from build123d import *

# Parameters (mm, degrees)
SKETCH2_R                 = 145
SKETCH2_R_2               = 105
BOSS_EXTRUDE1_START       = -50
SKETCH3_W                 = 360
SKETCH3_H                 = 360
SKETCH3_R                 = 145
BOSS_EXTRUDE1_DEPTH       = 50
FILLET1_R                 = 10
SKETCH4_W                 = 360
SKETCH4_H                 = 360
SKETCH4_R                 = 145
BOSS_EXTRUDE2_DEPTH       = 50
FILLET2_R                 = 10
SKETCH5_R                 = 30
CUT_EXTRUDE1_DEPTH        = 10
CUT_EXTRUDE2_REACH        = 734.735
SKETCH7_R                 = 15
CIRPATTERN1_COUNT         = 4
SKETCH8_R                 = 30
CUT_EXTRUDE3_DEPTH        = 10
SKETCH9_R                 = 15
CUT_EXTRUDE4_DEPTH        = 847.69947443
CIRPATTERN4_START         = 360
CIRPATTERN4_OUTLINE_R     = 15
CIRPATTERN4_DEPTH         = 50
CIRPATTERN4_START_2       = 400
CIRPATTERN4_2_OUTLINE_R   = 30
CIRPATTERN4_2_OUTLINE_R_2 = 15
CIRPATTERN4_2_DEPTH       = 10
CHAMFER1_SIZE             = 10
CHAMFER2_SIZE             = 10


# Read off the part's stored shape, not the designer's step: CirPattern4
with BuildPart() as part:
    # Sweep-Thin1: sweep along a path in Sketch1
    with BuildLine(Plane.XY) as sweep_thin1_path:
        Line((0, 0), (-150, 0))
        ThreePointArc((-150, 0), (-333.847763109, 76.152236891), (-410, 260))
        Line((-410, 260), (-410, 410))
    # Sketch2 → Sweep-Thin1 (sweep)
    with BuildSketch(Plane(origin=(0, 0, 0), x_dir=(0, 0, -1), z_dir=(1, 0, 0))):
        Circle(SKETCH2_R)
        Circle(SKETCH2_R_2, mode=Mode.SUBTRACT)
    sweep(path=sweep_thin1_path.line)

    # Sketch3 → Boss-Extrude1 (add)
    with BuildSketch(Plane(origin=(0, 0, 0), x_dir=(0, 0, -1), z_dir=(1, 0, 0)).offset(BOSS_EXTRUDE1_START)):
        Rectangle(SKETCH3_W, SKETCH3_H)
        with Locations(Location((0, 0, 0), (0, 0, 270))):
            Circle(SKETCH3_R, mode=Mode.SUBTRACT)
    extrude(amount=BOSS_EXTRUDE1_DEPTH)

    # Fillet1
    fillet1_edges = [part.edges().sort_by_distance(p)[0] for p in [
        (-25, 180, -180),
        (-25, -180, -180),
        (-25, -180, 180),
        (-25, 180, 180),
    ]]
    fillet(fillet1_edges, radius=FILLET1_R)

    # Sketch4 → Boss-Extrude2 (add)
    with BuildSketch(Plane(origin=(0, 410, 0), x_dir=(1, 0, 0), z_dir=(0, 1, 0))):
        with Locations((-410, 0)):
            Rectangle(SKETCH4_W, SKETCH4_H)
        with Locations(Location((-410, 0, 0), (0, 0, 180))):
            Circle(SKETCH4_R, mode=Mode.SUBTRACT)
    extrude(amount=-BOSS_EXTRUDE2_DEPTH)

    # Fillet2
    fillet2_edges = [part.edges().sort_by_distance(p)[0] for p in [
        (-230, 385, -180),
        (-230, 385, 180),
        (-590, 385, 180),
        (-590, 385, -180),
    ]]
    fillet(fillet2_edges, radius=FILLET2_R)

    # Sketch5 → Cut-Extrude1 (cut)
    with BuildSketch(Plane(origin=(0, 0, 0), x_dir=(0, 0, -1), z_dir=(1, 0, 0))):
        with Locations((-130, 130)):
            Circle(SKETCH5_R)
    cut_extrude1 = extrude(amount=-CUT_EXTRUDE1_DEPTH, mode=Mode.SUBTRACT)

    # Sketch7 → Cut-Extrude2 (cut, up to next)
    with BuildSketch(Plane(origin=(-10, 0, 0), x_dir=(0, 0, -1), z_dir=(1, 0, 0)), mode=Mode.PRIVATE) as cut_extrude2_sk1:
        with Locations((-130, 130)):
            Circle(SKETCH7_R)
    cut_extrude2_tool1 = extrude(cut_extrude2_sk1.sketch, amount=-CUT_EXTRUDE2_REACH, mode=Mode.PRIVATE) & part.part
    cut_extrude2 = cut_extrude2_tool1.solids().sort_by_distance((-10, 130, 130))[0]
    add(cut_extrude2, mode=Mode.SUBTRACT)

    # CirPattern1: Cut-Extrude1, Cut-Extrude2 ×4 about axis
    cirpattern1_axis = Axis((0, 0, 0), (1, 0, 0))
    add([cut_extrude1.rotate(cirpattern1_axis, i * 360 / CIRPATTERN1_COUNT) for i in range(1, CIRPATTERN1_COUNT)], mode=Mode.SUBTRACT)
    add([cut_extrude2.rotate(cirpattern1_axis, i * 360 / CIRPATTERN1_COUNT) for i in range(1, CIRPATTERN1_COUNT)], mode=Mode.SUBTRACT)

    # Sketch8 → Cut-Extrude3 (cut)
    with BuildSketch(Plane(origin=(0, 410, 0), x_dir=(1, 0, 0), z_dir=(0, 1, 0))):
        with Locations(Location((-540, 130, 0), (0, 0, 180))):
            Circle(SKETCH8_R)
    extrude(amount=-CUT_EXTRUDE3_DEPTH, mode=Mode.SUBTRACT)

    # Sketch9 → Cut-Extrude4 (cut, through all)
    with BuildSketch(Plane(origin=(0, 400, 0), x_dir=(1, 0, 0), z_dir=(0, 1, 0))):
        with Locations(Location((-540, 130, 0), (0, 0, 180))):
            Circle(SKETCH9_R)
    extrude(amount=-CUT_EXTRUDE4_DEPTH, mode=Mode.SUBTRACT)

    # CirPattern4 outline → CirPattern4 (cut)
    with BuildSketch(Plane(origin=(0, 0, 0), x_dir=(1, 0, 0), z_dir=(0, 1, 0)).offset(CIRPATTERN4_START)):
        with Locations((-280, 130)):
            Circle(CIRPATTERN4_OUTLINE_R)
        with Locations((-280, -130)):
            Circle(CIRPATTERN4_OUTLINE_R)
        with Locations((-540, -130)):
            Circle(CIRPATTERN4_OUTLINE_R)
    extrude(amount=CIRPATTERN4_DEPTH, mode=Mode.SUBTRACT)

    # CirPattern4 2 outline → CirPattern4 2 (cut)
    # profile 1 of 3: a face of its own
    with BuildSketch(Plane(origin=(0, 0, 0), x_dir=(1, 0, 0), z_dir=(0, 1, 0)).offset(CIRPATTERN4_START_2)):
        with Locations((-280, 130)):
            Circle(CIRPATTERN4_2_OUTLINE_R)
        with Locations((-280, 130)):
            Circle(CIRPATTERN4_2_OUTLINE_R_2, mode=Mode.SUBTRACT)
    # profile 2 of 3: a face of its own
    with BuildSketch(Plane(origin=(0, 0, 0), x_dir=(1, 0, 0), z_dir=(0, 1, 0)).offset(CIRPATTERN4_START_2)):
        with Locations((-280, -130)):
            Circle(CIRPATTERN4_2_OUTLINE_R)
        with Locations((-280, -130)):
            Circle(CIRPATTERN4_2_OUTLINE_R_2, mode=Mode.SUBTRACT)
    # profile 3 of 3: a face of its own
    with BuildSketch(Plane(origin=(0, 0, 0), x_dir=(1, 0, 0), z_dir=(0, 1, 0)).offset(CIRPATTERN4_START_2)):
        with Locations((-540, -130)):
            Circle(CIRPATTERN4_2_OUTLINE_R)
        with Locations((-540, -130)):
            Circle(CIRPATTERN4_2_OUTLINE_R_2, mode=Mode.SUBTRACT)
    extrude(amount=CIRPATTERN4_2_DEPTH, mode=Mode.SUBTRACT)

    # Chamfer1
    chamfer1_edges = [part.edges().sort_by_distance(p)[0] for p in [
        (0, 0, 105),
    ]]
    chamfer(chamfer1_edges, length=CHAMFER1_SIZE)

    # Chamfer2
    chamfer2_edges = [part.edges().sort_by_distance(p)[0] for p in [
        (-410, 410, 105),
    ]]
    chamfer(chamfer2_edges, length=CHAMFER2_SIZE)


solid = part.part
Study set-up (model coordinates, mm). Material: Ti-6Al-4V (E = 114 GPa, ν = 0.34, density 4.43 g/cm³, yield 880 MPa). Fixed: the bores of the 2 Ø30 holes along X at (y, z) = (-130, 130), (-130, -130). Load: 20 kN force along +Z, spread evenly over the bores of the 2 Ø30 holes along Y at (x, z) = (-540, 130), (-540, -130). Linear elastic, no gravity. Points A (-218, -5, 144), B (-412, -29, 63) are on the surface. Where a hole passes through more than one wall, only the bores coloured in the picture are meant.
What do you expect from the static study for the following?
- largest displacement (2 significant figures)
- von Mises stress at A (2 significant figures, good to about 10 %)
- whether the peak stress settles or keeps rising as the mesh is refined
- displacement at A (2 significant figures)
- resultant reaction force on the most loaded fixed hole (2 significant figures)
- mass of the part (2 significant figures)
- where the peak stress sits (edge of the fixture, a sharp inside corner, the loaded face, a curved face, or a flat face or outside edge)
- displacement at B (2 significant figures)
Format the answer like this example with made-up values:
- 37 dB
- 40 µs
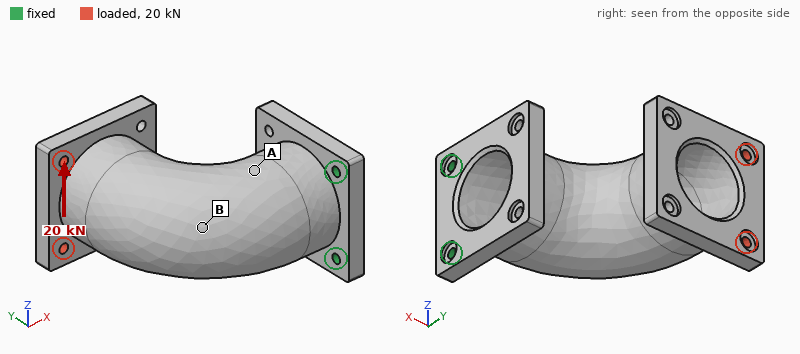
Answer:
- 0.30 mm
- 5.0 MPa
- keeps rising
- 0.081 mm
- 56 kN
- 120 kg
- edge of the fixture
- 0.12 mm
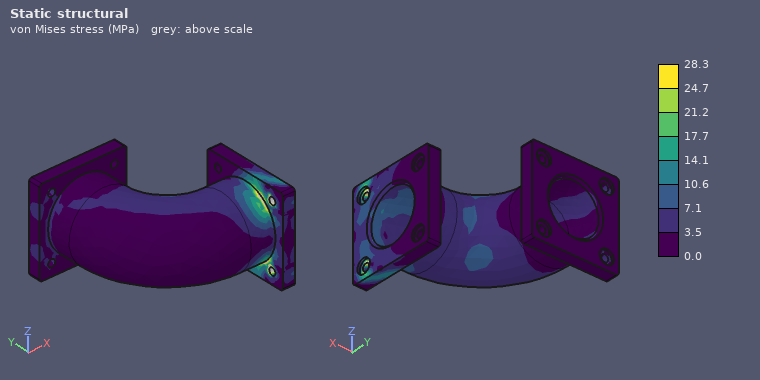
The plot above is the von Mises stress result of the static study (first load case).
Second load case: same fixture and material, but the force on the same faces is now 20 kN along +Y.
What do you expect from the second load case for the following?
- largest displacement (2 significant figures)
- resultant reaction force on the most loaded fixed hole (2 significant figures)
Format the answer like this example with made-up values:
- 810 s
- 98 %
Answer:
- 1.9 mm
- 10 kN
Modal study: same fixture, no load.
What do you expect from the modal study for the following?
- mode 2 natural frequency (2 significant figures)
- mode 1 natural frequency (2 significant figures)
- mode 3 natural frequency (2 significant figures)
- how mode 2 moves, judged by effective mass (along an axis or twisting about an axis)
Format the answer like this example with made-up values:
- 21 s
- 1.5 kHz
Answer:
- 220 Hz
- 69 Hz
- 540 Hz
- along Z
